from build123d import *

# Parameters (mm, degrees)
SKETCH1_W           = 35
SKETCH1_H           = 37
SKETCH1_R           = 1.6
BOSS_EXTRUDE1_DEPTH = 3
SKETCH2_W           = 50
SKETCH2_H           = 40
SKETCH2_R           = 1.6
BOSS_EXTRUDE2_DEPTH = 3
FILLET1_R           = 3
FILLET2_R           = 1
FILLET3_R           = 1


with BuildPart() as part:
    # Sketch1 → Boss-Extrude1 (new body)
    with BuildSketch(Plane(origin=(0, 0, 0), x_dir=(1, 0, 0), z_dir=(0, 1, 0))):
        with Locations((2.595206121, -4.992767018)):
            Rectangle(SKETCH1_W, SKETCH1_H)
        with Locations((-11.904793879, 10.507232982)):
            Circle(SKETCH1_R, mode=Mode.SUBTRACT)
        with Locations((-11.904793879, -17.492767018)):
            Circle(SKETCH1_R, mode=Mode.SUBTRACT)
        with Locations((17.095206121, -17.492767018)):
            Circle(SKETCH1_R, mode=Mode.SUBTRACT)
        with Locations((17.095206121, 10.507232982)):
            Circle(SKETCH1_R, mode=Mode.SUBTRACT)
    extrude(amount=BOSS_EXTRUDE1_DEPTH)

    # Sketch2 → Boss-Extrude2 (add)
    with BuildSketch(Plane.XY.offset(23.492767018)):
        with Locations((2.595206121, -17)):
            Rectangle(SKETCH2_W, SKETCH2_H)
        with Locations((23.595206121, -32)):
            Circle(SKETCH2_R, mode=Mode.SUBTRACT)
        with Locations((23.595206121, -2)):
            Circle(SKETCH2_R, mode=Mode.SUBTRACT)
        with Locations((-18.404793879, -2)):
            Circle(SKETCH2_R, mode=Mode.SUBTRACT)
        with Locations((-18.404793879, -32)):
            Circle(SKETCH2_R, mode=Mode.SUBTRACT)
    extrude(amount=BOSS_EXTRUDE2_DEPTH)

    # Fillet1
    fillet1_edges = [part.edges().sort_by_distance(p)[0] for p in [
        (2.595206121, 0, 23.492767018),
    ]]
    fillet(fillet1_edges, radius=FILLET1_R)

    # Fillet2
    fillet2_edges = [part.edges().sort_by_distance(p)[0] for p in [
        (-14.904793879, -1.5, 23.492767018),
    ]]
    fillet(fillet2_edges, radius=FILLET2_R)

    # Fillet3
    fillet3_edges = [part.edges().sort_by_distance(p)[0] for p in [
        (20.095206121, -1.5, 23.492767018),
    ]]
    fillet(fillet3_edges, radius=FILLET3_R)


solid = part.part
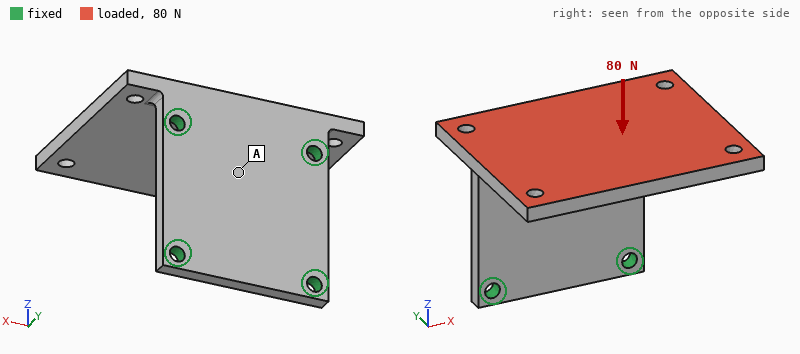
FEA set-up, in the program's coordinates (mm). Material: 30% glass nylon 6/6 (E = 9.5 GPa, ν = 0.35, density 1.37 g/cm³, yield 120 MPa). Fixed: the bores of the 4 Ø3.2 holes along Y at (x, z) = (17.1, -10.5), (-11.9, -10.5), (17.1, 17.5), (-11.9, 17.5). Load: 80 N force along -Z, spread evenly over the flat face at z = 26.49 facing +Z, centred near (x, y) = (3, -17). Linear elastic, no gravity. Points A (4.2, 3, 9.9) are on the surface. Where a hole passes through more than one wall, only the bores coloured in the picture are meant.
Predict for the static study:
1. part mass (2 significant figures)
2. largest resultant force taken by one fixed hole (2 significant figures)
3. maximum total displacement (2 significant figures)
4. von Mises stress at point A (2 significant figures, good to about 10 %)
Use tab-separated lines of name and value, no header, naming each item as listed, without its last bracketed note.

part mass	13 g
largest resultant force taken by one fixed hole	32 N
maximum total displacement	0.85 mm
von Mises stress at point A	4.8 MPa
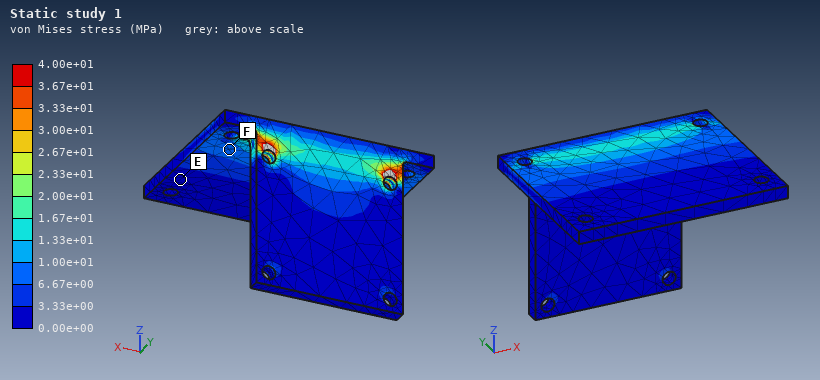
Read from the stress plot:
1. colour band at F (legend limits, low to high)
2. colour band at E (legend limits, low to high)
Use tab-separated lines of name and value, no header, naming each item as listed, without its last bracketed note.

colour band at F	6.67e+00 to 1.00e+01 MPa
colour band at E	0.00e+00 to 3.33e+00 MPa
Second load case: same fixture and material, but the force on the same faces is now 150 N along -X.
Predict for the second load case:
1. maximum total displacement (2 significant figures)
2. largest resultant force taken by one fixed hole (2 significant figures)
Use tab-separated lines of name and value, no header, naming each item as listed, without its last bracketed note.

maximum total displacement	96 µm
largest resultant force taken by one fixed hole	130 N
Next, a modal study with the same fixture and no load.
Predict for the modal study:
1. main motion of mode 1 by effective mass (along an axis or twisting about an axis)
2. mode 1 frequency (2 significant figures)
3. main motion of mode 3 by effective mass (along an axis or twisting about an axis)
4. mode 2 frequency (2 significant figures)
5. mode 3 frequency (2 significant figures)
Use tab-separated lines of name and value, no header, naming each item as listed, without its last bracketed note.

main motion of mode 1 by effective mass	along Z
mode 1 frequency	670 Hz
main motion of mode 3 by effective mass	along X
mode 2 frequency	1400 Hz
mode 3 frequency	2700 Hz
